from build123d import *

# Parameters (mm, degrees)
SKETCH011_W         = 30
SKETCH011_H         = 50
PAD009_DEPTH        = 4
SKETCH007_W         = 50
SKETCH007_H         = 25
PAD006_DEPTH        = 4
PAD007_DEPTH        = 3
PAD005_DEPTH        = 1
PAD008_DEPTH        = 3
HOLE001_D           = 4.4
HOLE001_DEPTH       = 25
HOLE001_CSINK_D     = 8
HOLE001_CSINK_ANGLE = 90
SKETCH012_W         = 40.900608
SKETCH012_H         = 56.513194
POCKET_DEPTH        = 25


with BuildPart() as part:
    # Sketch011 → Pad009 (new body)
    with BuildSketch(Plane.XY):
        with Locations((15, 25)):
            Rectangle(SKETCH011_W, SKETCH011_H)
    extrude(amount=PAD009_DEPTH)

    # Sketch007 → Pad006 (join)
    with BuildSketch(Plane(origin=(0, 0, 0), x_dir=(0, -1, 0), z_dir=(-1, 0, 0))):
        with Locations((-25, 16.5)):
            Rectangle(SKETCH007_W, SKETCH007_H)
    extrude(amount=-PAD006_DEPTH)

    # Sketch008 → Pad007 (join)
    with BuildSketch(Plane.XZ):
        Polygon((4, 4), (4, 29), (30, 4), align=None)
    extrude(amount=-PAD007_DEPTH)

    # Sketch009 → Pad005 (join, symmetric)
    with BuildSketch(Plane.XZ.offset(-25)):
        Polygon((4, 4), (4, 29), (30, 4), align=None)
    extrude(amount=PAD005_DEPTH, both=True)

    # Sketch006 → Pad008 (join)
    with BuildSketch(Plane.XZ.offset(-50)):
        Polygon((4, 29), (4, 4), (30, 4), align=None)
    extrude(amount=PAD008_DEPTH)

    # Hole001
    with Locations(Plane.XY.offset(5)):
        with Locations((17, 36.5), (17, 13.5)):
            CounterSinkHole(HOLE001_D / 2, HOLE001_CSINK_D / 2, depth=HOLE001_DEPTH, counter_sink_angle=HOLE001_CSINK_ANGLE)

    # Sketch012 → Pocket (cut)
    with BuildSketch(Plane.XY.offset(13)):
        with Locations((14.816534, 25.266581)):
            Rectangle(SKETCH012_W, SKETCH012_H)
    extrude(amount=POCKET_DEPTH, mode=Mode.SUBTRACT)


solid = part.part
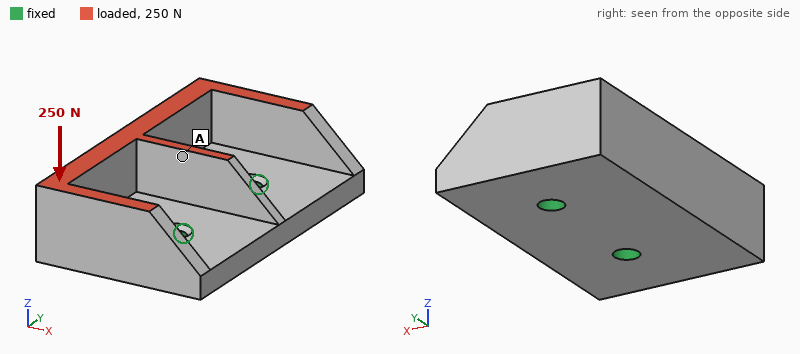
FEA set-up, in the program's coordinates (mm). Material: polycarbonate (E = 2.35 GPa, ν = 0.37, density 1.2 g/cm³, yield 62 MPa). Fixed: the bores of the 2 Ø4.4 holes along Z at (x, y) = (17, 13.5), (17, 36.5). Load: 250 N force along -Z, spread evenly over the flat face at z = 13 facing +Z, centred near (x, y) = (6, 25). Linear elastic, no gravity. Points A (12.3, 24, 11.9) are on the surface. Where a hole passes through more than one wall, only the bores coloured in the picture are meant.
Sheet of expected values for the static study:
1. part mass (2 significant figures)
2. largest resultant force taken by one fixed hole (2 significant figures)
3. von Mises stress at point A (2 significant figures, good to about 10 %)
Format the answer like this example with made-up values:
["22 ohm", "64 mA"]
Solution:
["11 g", "130 N", "5.0 MPa"]
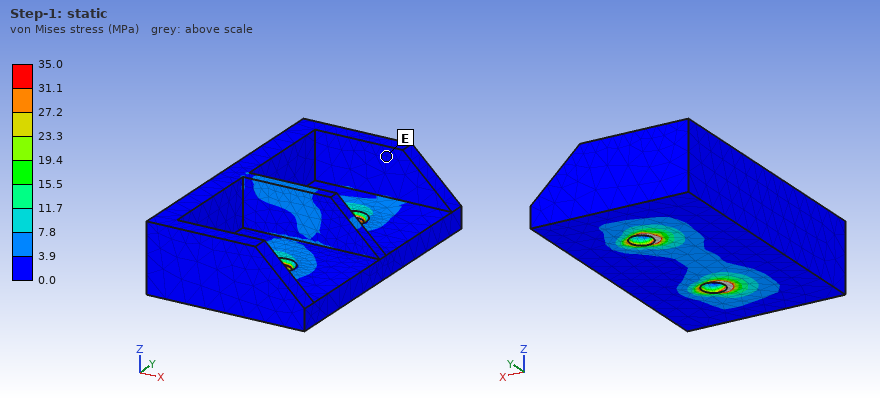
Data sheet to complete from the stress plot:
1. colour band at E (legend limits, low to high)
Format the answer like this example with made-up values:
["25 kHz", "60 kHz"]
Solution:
["0.0 to 3.9 MPa"]
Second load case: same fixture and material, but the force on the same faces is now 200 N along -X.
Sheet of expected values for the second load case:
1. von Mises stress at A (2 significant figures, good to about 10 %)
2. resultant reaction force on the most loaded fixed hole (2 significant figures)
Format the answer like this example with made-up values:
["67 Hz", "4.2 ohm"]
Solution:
["6.2 MPa", "100 N"]
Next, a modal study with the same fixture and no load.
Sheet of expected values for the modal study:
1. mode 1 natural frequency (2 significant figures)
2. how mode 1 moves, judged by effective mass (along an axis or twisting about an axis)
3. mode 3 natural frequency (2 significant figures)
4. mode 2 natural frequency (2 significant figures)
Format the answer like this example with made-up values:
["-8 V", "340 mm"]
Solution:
["1700 Hz", "along Z", "3200 Hz", "1900 Hz"]
